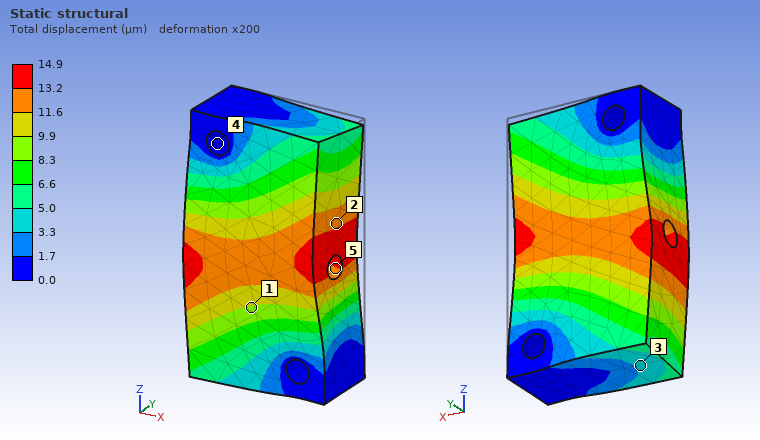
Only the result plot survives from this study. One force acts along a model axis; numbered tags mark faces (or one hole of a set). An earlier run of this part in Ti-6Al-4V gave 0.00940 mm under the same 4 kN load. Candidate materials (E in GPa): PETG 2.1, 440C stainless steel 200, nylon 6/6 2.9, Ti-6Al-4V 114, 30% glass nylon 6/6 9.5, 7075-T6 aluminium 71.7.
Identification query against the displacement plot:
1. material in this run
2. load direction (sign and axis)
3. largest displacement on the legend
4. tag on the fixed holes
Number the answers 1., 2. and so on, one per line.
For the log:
1. 7075-T6 aluminium
2. -Y
3. 14.9 µm
4. 4
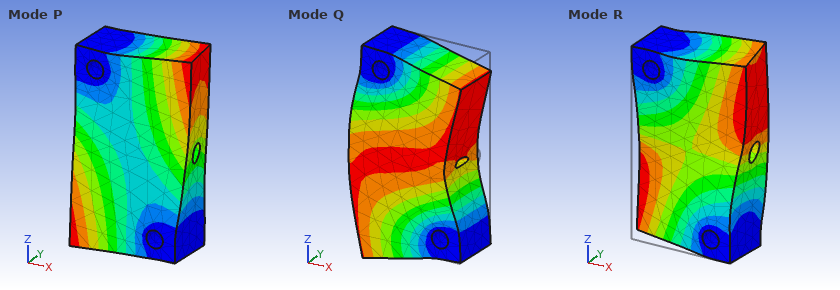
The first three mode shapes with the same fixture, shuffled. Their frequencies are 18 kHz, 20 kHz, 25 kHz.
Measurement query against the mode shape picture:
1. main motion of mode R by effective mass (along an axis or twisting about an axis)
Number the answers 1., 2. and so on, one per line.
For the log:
1. along Y
